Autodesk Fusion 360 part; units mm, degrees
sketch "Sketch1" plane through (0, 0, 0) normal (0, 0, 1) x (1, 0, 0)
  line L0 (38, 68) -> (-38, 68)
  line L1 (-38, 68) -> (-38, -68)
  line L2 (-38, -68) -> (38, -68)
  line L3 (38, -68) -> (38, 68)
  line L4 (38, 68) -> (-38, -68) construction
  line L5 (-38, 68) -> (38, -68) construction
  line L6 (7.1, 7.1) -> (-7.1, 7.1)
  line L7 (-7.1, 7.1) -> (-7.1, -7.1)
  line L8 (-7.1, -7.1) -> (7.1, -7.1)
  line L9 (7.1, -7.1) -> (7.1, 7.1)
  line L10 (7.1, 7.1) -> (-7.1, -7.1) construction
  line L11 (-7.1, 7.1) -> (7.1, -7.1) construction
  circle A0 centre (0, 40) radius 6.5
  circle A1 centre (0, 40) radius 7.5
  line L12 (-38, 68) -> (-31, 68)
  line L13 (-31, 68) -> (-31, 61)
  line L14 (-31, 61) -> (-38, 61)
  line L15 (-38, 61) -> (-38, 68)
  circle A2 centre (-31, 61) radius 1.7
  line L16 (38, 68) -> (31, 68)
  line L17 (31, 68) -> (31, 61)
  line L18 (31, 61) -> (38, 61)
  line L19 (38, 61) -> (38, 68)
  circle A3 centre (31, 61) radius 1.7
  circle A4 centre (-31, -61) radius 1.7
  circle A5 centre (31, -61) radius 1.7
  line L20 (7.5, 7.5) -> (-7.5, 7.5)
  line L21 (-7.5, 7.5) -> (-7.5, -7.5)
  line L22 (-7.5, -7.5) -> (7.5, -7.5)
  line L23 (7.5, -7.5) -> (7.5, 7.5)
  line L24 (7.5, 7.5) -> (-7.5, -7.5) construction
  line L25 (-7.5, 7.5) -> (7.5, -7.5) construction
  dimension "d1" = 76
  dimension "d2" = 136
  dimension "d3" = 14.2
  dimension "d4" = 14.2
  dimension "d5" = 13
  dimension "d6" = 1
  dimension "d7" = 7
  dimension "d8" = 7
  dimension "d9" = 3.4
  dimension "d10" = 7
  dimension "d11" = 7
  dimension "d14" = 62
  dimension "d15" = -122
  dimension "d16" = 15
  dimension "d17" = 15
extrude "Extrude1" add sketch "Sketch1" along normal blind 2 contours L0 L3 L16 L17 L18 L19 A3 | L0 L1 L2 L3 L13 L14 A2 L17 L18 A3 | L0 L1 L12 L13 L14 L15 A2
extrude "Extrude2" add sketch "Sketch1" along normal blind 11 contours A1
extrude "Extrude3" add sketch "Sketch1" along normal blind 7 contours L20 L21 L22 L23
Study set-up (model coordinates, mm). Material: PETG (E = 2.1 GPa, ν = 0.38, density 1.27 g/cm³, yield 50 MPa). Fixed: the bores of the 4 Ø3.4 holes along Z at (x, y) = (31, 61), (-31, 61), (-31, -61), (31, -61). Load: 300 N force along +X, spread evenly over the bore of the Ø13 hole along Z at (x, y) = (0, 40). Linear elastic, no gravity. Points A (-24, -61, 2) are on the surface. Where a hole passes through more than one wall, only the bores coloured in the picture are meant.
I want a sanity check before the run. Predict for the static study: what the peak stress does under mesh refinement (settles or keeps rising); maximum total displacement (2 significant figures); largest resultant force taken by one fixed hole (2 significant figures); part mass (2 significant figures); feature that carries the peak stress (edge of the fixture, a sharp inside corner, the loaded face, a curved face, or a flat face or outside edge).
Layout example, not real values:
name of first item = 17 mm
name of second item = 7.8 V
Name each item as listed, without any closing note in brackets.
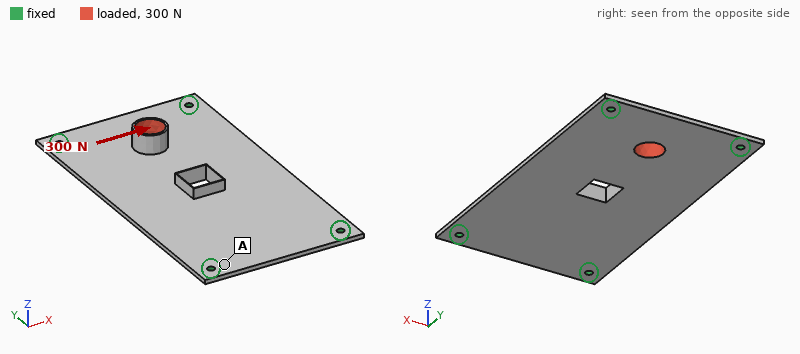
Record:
what the peak stress does under mesh refinement = keeps rising
maximum total displacement = 1.4 mm
largest resultant force taken by one fixed hole = 140 N
part mass = 26 g
feature that carries the peak stress = edge of the fixture
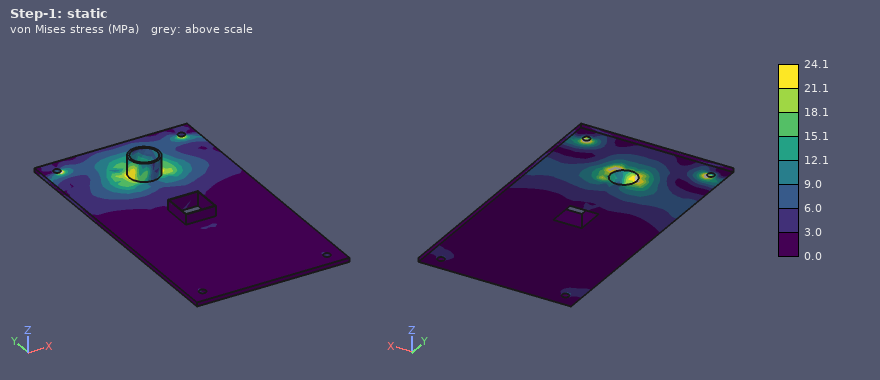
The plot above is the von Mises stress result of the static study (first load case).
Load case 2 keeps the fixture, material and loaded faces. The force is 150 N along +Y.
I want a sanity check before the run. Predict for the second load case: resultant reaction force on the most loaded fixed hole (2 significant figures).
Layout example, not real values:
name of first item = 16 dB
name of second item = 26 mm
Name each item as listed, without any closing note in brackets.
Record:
resultant reaction force on the most loaded fixed hole = 55 N
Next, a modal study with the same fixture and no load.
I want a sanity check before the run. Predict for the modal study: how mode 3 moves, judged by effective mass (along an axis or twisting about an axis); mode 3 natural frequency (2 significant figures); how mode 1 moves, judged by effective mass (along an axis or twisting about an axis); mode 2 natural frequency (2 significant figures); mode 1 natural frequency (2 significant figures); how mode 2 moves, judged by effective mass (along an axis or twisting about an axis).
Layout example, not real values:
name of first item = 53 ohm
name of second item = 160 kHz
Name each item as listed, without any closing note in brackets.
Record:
how mode 3 moves, judged by effective mass = twisting about X
mode 3 natural frequency = 430 Hz
how mode 1 moves, judged by effective mass = along Z
mode 2 natural frequency = 260 Hz
mode 1 natural frequency = 160 Hz
how mode 2 moves, judged by effective mass = twisting about Y
